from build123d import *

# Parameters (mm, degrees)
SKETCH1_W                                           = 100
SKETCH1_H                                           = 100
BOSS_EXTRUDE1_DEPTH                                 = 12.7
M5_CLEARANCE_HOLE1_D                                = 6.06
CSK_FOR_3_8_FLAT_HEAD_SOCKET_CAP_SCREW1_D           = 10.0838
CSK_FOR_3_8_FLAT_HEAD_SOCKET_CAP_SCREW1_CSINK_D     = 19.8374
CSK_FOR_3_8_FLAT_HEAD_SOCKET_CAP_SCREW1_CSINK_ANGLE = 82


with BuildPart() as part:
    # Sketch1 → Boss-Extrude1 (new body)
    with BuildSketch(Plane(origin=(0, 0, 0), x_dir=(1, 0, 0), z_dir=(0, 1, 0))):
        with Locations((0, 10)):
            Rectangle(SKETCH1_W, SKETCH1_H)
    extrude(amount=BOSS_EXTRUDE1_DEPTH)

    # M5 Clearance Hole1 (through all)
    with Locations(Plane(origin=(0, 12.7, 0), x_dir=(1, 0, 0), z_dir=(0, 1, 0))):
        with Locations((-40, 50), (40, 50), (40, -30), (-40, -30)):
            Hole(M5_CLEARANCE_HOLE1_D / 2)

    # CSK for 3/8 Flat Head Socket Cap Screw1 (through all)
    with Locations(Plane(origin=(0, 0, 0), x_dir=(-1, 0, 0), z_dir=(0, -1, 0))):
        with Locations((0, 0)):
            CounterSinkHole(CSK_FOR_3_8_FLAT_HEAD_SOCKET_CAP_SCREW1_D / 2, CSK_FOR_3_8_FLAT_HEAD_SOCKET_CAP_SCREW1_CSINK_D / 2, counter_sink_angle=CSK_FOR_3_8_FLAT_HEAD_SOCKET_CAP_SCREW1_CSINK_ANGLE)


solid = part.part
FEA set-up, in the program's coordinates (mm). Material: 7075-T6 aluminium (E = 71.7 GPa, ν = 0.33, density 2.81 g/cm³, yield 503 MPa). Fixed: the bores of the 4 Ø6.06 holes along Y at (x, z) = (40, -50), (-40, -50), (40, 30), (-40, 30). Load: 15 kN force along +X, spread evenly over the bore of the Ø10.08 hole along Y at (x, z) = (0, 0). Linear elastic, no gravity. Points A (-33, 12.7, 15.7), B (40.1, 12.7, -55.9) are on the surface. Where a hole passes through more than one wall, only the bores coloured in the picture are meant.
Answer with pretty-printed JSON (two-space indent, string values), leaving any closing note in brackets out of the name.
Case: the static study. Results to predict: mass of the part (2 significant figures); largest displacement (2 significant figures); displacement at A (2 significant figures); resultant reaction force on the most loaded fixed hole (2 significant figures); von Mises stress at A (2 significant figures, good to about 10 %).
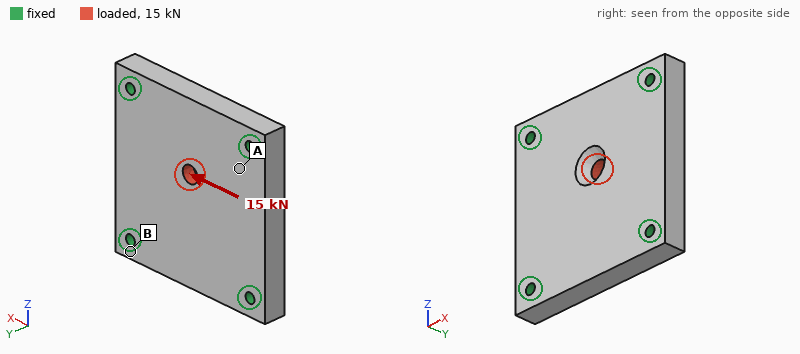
{
  "mass of the part": "350 g",
  "largest displacement": "20 µm",
  "displacement at A": "5.9 µm",
  "resultant reaction force on the most loaded fixed hole": "4.9 kN",
  "von Mises stress at A": "15 MPa"
}
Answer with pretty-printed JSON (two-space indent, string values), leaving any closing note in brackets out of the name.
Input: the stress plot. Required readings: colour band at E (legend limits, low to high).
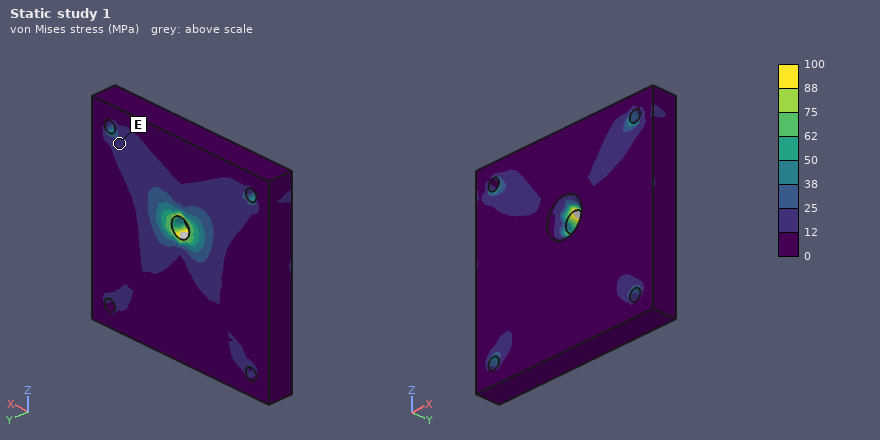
{
  "colour band at E": "12 to 25 MPa"
}
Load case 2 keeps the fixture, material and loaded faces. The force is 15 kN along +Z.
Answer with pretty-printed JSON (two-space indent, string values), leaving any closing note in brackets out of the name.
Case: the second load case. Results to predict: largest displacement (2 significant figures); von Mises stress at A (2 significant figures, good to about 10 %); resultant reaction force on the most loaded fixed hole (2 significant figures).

{
  "largest displacement": "22 µm",
  "von Mises stress at A": "16 MPa",
  "resultant reaction force on the most loaded fixed hole": "4.4 kN"
}
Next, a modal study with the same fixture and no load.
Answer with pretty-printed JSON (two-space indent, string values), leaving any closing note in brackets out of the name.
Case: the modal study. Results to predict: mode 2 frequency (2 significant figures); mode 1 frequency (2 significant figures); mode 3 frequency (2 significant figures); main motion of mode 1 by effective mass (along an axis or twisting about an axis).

{
  "mode 2 frequency": "9400 Hz",
  "mode 1 frequency": "5900 Hz",
  "mode 3 frequency": "9400 Hz",
  "main motion of mode 1 by effective mass": "along Y"
}
